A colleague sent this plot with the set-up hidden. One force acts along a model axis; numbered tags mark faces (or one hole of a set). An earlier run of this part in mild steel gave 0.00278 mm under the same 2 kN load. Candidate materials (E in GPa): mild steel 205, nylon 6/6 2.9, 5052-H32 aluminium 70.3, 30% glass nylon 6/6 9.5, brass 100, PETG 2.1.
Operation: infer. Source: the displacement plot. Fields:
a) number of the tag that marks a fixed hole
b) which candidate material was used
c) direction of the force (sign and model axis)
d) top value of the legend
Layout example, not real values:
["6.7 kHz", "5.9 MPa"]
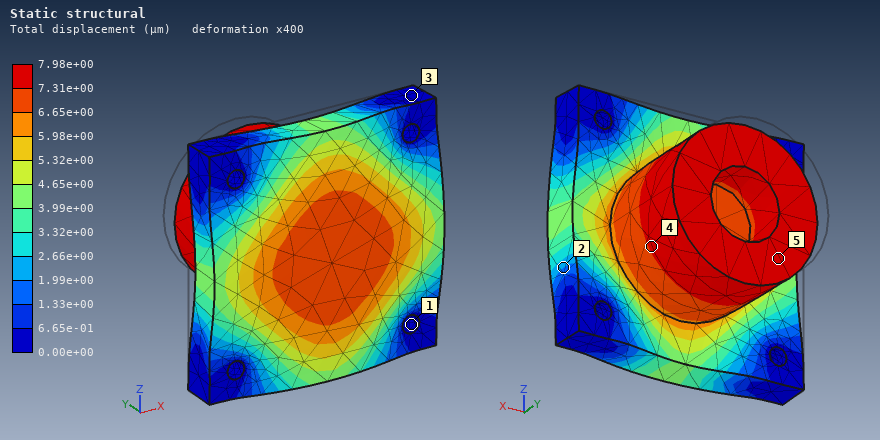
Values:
["1", "5052-H32 aluminium", "-Y", "7.98e+00 µm"]
